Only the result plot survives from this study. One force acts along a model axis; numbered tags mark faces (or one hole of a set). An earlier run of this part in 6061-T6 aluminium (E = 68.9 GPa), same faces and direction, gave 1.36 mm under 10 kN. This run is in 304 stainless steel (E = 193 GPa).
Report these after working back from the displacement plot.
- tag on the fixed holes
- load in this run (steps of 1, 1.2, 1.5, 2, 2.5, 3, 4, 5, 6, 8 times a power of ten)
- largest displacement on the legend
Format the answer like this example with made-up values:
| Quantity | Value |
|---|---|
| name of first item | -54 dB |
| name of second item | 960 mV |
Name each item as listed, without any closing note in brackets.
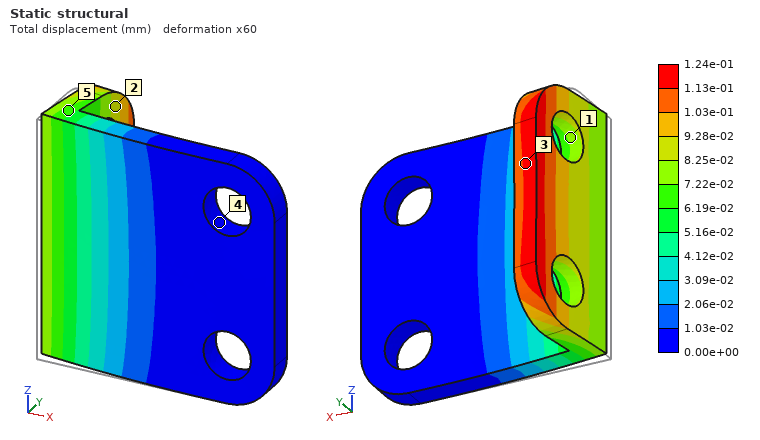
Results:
| Quantity | Value |
|---|---|
| tag on the fixed holes | 4 |
| load in this run | 2.5 kN |
| largest displacement on the legend | 1.24e-01 mm |
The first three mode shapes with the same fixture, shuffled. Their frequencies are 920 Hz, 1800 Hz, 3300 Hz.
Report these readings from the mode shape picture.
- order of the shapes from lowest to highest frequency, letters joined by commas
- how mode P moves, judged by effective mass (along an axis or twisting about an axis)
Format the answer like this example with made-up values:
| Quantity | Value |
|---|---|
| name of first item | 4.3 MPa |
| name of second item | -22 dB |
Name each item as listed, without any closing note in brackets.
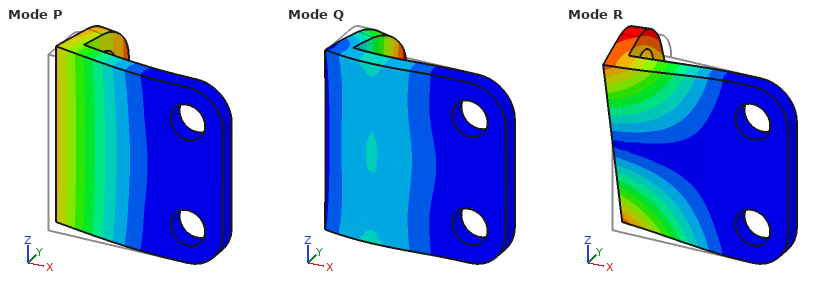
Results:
| Quantity | Value |
|---|---|
| order of the shapes from lowest to highest frequency, letters joined by commas | P, R, Q |
| how mode P moves, judged by effective mass | along Y |
